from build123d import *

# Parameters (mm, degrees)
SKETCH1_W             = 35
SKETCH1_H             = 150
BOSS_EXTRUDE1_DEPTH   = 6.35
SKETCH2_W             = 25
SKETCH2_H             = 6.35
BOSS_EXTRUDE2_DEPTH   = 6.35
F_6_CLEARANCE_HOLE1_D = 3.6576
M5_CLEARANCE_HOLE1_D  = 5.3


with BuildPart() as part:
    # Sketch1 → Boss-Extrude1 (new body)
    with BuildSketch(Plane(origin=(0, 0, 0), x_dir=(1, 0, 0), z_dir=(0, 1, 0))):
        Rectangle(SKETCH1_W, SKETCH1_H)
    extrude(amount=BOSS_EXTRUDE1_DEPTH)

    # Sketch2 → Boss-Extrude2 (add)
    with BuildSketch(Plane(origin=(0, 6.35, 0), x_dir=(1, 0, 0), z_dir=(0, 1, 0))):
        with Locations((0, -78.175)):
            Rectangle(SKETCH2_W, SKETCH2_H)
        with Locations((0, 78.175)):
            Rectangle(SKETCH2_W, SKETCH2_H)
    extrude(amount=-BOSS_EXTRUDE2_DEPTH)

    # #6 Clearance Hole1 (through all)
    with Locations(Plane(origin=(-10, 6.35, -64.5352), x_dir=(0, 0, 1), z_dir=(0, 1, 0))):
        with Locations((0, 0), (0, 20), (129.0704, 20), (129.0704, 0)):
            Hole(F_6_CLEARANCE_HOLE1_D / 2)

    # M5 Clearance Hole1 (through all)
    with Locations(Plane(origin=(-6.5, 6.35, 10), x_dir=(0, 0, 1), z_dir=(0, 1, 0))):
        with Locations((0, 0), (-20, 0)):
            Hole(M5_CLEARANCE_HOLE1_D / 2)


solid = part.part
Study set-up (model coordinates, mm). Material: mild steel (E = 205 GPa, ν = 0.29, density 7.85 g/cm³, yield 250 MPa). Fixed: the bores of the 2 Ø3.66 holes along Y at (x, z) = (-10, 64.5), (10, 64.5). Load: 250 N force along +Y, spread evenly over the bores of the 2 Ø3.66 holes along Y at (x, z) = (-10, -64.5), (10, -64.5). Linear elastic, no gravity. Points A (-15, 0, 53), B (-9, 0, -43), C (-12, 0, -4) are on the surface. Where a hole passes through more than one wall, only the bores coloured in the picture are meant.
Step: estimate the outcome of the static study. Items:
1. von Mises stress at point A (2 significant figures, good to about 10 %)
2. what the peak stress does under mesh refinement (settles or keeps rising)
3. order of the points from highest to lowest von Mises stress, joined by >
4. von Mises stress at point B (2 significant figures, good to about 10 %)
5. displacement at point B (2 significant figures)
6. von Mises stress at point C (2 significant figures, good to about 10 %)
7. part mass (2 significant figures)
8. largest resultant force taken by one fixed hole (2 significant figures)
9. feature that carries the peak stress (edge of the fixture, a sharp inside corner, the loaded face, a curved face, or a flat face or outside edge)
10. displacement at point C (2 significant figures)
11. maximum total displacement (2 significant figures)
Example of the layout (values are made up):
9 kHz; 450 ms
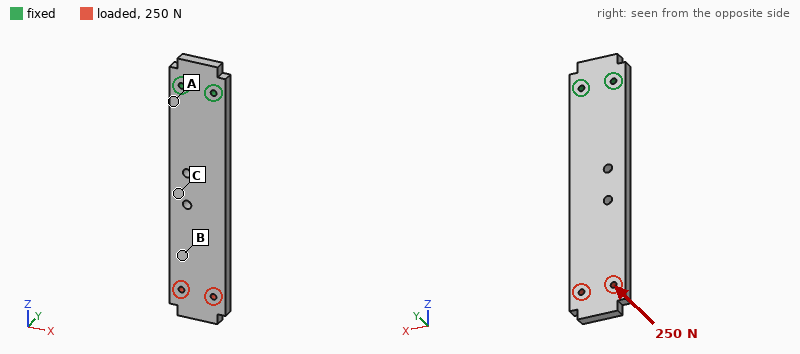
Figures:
130 MPa; keeps rising; A > C > B; 23 MPa; 0.90 mm; 67 MPa; 270 g; 130 N; edge of the fixture; 0.42 mm; 1.4 mm
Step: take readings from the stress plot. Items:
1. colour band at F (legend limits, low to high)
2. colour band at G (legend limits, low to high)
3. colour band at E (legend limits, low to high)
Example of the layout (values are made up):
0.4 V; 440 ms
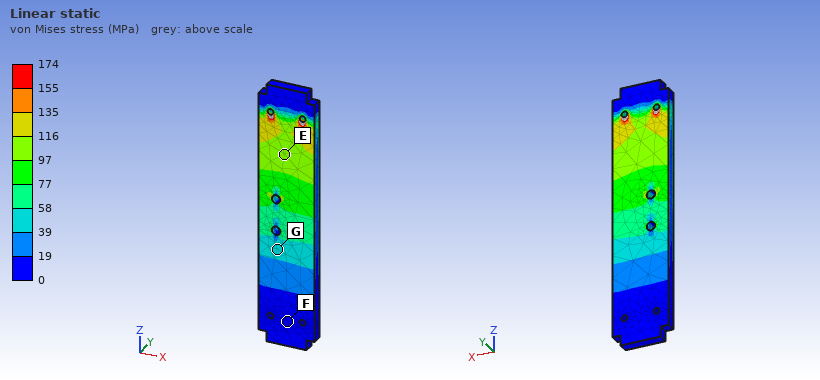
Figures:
0 to 19 MPa; 39 to 58 MPa; 97 to 116 MPa
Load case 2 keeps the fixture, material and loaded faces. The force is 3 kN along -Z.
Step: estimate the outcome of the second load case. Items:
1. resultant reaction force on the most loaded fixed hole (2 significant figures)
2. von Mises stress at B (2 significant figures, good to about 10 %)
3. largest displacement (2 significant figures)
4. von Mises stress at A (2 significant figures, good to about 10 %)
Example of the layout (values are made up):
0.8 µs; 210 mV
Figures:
1.5 kN; 14 MPa; 9.6 µm; 13 MPa
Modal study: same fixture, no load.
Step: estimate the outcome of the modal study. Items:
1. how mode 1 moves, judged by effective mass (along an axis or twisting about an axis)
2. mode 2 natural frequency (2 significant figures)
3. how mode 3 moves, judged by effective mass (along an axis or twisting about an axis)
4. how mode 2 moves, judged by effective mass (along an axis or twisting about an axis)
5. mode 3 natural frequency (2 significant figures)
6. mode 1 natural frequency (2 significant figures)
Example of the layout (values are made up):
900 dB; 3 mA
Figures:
along Y; 1300 Hz; along Y; along X; 1500 Hz; 250 Hz
